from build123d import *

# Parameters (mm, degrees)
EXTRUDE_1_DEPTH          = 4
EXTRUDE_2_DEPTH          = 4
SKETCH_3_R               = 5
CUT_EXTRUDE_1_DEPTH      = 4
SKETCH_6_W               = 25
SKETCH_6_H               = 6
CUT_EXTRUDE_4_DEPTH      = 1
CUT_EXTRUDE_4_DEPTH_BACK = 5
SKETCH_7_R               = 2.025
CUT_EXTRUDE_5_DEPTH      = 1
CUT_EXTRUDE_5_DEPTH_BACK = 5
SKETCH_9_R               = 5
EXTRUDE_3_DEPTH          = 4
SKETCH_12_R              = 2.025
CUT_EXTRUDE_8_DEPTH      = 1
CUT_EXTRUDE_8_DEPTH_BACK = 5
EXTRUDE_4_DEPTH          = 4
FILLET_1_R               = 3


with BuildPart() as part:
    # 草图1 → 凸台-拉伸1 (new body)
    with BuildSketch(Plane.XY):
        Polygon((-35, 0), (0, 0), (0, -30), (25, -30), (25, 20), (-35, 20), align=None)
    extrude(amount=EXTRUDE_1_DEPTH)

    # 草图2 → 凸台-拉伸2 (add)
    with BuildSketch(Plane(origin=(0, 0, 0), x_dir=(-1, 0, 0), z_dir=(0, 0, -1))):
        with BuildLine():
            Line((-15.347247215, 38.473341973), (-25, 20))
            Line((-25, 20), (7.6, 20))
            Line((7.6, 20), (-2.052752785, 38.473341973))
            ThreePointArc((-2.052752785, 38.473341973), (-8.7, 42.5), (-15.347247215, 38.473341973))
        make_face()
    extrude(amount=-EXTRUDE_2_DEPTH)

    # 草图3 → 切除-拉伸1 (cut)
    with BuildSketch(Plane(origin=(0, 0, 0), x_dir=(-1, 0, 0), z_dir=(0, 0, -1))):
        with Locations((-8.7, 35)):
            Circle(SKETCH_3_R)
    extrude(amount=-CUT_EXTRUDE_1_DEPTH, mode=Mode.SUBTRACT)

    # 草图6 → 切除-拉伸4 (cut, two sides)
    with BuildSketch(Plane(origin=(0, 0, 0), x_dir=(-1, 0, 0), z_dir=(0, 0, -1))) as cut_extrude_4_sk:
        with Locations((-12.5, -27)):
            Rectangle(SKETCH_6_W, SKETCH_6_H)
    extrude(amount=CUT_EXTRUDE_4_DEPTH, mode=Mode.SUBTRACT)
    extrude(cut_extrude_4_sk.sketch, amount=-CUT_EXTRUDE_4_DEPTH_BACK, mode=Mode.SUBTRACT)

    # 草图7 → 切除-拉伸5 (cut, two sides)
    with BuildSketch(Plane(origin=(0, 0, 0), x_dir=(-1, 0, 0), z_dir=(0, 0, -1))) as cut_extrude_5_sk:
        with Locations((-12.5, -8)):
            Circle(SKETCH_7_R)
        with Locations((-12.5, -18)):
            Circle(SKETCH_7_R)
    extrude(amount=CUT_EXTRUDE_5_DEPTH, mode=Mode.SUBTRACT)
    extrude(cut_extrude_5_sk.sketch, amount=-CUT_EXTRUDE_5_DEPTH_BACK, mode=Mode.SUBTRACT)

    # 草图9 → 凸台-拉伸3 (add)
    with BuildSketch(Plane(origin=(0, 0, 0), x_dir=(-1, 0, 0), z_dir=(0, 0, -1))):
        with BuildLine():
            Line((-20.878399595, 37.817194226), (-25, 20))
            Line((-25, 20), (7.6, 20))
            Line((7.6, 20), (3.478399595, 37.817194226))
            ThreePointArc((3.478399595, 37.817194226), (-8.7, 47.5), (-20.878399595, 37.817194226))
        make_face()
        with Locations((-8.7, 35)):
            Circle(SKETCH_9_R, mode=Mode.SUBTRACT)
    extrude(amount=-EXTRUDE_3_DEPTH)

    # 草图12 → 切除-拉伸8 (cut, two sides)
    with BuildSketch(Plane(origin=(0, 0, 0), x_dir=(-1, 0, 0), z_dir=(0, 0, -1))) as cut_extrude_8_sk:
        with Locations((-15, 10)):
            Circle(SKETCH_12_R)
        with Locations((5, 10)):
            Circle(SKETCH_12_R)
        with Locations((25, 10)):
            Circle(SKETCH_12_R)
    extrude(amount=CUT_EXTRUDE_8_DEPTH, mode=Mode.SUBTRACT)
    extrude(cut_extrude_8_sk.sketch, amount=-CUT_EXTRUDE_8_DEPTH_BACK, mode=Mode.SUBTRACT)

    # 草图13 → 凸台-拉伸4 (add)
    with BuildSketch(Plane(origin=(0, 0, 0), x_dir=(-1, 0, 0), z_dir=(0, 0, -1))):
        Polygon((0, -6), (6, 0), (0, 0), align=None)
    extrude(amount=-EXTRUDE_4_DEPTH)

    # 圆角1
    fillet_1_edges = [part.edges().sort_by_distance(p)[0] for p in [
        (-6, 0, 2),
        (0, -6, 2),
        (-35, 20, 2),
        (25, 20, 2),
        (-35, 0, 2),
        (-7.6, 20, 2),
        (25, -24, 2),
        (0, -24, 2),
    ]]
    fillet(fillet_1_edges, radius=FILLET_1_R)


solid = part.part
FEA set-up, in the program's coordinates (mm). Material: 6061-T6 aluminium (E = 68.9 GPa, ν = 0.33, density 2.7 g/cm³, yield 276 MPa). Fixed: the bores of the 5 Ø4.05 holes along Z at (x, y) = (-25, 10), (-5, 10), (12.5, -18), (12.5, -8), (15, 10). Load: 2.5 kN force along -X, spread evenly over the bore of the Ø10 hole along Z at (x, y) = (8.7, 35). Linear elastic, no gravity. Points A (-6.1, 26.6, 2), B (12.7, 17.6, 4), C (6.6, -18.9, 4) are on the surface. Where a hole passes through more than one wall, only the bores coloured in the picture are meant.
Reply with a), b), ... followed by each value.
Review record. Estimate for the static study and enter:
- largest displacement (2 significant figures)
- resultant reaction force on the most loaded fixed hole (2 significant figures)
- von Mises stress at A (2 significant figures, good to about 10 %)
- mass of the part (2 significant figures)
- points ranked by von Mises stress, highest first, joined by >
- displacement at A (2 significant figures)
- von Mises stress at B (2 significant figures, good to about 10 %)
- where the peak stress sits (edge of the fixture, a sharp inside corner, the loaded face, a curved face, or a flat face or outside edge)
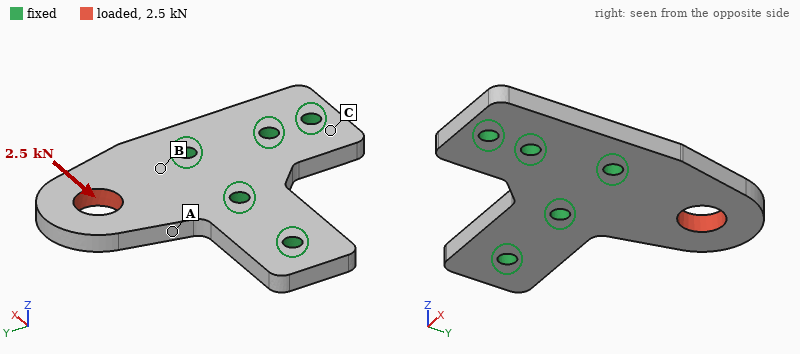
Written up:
a) 57 µm
b) 2.2 kN
c) 65 MPa
d) 25 g
e) A > B > C
f) 22 µm
g) 41 MPa
h) a curved face
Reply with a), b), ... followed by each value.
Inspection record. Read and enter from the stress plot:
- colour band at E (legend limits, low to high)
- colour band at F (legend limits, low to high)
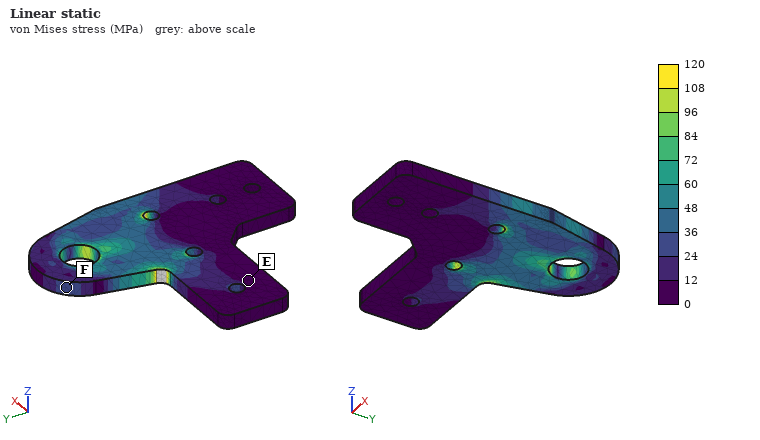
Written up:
a) 0 to 12 MPa
b) 24 to 36 MPa
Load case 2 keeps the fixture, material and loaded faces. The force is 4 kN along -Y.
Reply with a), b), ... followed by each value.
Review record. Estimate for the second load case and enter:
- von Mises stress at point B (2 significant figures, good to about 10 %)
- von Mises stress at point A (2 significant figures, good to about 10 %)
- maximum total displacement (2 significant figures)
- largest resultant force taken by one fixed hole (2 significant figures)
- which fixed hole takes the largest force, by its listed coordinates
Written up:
a) 43 MPa
b) 31 MPa
c) 23 µm
d) 2.2 kN
e) (15, 10)
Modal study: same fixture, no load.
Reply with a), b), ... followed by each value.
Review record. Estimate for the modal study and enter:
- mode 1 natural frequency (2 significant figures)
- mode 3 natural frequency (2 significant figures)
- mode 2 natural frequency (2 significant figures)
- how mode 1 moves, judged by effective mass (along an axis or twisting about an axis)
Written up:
a) 3300 Hz
b) 14 kHz
c) 9300 Hz
d) along Z
